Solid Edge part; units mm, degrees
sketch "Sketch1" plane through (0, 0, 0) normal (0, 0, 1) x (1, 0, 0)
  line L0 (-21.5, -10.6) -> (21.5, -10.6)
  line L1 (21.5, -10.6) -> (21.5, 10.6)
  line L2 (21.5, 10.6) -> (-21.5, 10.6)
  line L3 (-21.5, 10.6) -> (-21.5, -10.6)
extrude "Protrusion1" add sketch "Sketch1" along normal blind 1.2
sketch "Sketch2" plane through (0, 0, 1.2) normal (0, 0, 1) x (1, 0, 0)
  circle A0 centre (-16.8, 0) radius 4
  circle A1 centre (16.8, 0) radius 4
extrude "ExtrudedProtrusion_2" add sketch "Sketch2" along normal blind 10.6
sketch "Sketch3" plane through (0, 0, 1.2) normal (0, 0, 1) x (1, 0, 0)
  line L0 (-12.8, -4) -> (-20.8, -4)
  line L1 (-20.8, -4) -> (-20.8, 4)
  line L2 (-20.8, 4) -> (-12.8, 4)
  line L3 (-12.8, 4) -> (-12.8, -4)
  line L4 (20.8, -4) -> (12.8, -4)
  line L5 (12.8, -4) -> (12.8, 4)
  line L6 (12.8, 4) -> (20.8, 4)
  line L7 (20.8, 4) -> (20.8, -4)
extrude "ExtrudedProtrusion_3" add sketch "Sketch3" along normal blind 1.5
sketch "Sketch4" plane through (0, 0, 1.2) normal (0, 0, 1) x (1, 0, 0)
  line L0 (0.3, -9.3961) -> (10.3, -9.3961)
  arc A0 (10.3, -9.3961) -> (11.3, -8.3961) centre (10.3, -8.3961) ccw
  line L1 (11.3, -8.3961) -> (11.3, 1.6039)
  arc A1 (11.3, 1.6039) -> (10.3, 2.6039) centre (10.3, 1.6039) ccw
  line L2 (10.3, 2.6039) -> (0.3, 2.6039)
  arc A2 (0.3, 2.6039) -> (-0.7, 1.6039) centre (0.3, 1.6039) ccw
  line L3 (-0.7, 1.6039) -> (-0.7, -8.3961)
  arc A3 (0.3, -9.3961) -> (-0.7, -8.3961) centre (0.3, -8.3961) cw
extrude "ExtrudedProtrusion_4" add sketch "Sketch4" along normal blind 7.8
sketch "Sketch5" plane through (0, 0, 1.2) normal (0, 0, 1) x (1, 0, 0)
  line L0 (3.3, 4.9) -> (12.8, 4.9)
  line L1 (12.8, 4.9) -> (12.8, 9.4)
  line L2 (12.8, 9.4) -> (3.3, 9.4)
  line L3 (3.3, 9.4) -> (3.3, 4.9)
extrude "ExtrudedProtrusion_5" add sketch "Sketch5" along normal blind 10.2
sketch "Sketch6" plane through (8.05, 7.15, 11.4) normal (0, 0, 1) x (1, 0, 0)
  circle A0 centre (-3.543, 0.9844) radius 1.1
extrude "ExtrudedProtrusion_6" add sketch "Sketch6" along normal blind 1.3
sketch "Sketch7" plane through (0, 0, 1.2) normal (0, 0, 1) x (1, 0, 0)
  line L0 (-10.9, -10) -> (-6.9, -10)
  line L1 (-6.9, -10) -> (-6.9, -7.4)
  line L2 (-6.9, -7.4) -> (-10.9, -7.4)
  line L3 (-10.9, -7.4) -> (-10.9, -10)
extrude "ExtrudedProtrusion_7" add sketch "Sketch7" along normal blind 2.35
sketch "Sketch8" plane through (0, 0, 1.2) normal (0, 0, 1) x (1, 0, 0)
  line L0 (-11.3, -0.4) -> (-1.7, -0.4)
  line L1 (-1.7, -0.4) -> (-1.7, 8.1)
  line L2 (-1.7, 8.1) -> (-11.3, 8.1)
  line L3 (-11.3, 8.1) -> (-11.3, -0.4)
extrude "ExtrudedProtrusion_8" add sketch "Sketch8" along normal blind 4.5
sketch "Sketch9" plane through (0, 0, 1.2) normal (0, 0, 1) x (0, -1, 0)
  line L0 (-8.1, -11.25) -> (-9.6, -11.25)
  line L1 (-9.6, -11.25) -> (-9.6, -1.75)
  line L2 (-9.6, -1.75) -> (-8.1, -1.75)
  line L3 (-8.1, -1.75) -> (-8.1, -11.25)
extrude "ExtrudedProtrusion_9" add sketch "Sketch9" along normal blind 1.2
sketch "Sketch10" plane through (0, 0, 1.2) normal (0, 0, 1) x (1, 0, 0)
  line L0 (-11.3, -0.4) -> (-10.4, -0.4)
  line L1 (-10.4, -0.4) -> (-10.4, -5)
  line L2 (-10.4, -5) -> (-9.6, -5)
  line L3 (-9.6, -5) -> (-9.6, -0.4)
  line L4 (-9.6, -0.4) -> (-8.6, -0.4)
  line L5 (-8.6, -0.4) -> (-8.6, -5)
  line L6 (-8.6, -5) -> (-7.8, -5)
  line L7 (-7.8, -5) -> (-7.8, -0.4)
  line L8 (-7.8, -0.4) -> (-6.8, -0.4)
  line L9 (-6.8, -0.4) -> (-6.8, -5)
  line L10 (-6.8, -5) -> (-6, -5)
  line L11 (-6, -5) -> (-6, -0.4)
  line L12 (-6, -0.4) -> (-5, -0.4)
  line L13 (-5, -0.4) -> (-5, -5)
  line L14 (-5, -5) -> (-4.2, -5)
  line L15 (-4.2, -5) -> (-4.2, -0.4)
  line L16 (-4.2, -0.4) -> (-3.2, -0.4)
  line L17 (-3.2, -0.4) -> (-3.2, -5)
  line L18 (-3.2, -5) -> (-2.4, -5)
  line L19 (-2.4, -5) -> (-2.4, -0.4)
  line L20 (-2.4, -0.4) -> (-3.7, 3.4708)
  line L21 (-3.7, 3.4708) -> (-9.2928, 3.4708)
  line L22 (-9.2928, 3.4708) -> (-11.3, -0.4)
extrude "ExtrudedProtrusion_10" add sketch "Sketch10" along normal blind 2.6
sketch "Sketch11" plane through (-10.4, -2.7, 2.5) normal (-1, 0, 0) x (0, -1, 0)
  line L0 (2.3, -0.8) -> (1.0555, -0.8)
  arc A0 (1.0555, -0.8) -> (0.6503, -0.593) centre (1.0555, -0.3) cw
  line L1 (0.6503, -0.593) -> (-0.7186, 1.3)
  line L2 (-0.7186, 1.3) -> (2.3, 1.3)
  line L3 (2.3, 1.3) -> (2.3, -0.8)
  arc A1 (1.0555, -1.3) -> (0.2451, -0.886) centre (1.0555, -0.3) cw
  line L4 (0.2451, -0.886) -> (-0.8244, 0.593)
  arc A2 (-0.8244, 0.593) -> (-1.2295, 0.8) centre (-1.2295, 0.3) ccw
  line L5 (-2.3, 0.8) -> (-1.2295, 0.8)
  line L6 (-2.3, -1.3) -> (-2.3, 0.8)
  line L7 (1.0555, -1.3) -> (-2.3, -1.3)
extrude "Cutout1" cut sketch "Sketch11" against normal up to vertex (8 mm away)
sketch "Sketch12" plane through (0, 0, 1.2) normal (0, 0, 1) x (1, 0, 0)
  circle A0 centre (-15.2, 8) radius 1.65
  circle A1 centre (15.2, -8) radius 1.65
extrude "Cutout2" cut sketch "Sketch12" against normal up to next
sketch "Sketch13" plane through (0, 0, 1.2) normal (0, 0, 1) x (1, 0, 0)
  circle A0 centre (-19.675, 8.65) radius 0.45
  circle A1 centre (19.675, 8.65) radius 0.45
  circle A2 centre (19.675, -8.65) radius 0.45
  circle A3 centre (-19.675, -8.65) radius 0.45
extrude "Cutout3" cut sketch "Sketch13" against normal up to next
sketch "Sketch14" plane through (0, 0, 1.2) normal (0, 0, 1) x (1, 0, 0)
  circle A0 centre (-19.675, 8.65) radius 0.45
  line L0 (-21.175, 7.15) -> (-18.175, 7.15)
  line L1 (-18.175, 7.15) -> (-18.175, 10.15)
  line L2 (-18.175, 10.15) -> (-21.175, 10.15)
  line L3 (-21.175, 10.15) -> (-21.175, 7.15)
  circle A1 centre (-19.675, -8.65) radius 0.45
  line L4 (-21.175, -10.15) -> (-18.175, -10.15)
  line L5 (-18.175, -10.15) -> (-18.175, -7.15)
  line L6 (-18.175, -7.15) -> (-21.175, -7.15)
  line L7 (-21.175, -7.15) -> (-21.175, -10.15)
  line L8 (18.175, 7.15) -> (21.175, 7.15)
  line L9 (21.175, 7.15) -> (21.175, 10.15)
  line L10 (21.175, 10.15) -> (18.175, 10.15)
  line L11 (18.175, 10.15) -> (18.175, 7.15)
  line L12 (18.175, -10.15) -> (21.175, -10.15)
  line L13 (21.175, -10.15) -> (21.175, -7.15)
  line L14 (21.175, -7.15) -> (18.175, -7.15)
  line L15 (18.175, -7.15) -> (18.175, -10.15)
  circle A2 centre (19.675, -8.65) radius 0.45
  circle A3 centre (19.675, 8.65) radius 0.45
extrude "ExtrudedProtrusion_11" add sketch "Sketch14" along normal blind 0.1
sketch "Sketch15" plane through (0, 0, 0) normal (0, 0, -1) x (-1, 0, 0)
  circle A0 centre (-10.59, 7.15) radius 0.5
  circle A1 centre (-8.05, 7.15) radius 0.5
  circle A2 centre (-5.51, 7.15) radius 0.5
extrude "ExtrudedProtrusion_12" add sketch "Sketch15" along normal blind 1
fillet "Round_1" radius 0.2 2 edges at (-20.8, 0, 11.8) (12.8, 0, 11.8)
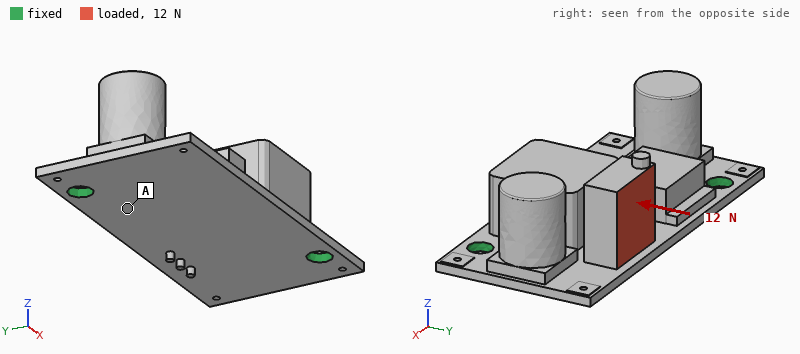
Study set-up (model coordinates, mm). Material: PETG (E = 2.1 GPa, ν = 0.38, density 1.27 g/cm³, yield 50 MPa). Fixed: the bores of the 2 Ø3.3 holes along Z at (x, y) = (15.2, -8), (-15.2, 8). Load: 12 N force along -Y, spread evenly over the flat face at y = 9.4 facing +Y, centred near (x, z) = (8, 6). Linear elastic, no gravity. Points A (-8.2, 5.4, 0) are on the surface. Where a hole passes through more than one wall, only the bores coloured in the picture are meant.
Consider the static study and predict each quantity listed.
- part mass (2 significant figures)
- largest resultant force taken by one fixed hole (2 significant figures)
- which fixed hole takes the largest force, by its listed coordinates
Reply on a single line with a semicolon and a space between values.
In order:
5.3 g; 8.7 N; (15.2, -8)
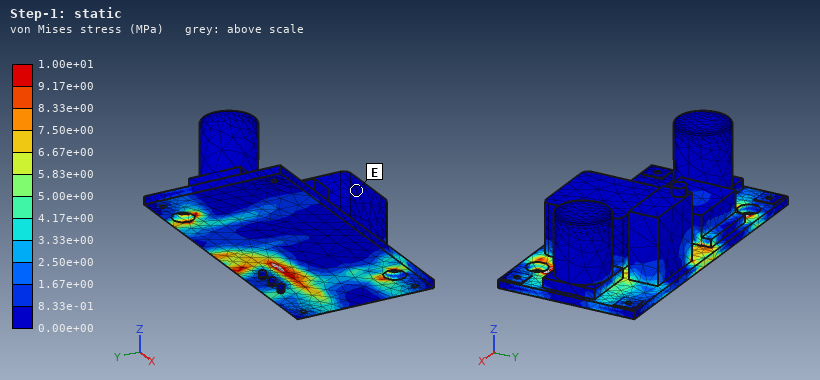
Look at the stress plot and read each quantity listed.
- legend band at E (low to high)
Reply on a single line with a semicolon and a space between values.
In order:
0.00e+00 to 8.33e-01 MPa
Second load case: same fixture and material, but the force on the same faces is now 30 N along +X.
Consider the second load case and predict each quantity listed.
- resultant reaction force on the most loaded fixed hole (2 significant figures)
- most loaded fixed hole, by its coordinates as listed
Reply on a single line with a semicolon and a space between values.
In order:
20 N; (-15.2, 8)
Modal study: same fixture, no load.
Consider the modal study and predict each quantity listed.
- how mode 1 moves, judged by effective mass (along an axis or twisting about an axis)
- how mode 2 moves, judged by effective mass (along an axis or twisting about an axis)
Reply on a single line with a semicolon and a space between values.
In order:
along Y; along Z
